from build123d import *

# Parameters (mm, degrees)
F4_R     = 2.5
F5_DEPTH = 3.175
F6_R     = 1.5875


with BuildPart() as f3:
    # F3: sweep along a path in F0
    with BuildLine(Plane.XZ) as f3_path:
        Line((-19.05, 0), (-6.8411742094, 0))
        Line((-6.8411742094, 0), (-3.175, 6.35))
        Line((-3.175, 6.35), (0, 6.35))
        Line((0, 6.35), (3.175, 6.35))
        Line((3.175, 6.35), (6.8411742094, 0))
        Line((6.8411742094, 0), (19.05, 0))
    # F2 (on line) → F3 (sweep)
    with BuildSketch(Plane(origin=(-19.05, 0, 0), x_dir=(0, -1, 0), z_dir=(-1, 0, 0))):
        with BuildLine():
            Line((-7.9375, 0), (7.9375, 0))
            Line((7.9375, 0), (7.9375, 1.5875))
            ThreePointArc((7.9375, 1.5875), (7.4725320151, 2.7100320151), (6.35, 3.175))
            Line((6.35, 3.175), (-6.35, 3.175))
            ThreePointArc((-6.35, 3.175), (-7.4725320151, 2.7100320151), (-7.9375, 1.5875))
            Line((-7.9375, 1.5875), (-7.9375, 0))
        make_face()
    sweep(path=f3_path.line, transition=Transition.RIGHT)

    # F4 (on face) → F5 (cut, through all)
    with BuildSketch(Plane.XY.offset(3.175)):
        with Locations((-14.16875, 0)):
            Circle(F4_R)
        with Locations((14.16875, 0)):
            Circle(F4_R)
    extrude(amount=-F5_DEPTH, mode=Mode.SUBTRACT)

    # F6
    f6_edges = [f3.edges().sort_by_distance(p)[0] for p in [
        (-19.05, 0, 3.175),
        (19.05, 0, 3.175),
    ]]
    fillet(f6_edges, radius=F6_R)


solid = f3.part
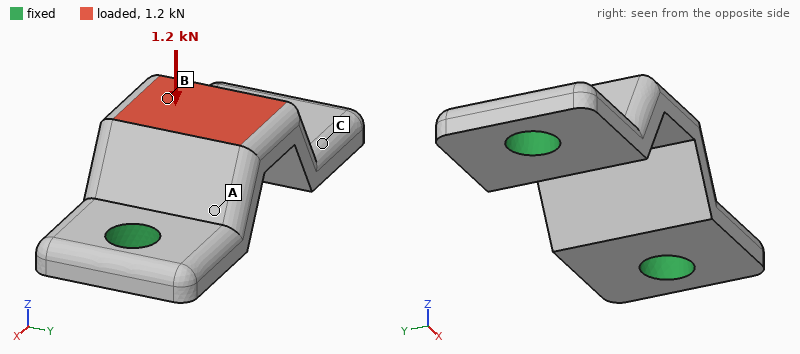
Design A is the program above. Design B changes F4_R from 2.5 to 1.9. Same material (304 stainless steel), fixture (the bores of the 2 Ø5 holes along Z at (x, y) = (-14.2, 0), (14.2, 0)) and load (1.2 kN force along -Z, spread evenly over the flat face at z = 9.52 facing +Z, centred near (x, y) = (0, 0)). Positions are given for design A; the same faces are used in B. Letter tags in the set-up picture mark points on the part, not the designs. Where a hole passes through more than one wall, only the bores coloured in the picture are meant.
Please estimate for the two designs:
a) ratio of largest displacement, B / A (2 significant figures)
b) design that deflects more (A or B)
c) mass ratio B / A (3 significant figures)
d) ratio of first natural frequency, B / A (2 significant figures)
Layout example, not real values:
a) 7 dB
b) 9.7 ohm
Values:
a) 1.2
b) B
c) 1.03
d) 0.86
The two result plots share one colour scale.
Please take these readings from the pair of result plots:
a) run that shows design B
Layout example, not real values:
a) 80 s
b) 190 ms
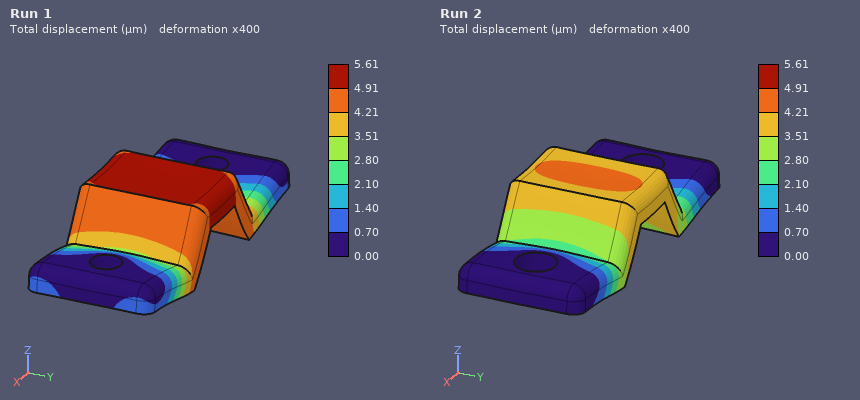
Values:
a) Run 1
